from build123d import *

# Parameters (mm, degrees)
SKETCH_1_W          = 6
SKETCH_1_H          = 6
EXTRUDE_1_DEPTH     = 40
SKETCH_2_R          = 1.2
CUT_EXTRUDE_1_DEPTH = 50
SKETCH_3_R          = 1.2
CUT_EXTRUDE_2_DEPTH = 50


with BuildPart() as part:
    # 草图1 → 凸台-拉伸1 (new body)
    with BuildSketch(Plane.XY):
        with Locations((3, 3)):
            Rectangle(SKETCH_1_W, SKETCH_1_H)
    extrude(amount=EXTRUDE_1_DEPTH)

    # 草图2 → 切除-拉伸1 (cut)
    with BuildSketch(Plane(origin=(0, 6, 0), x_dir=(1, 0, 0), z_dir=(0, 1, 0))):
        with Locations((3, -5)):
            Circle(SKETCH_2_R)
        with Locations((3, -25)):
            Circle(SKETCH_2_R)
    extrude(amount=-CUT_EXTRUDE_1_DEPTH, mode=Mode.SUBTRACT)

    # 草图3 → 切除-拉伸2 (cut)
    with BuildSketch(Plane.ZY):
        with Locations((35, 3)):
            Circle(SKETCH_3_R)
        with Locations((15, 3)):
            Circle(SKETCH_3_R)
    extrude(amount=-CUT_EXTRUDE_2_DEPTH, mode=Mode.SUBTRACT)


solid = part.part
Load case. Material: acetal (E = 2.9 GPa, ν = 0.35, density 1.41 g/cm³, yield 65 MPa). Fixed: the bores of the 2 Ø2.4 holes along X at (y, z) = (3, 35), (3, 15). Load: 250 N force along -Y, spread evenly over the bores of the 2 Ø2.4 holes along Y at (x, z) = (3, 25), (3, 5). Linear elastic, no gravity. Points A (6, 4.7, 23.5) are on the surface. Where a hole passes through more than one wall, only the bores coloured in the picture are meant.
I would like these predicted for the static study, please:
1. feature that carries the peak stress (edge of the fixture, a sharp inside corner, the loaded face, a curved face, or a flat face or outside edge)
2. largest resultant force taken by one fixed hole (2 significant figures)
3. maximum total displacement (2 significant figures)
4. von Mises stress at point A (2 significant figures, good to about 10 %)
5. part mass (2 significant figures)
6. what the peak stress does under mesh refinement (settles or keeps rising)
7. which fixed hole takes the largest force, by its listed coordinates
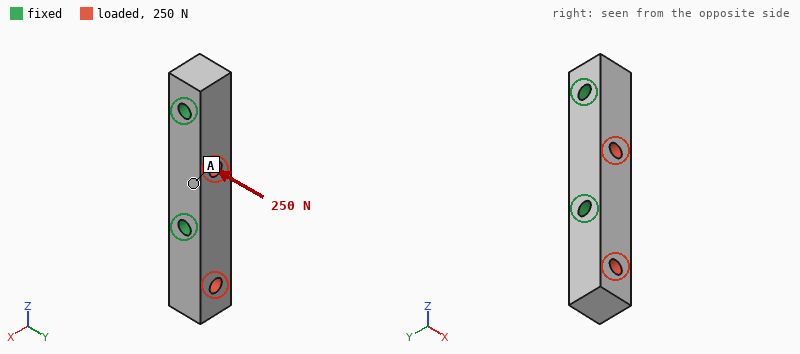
edge of the fixture
200 N
0.33 mm
4.7 MPa
1.9 g
keeps rising
(3, 15)
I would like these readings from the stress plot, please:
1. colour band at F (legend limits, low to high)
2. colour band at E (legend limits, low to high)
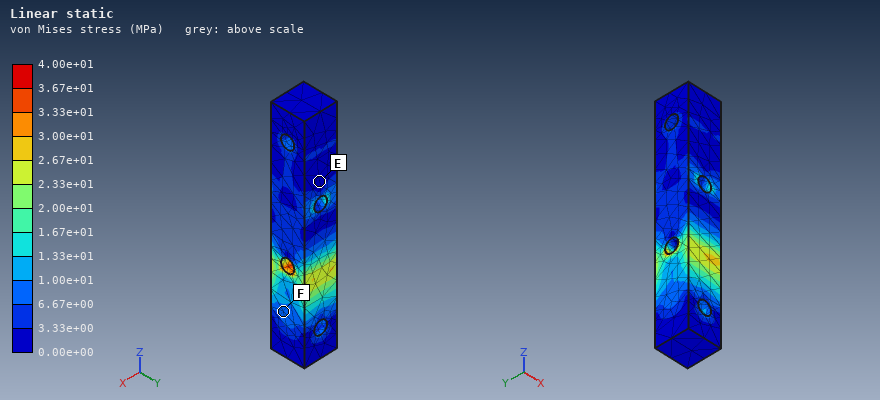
6.67e+00 to 1.00e+01 MPa
0.00e+00 to 3.33e+00 MPa
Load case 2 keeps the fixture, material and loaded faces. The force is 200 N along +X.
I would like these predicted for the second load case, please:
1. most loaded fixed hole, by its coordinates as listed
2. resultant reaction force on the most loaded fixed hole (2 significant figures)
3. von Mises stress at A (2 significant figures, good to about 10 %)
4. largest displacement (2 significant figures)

(3, 15)
150 N
4.4 MPa
0.21 mm
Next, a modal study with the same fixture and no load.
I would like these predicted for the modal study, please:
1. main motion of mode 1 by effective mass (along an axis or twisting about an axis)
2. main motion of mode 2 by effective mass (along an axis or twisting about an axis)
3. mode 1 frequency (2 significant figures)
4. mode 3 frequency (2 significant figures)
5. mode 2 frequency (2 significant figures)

along Y
along X
5100 Hz
14 kHz
5900 Hz
